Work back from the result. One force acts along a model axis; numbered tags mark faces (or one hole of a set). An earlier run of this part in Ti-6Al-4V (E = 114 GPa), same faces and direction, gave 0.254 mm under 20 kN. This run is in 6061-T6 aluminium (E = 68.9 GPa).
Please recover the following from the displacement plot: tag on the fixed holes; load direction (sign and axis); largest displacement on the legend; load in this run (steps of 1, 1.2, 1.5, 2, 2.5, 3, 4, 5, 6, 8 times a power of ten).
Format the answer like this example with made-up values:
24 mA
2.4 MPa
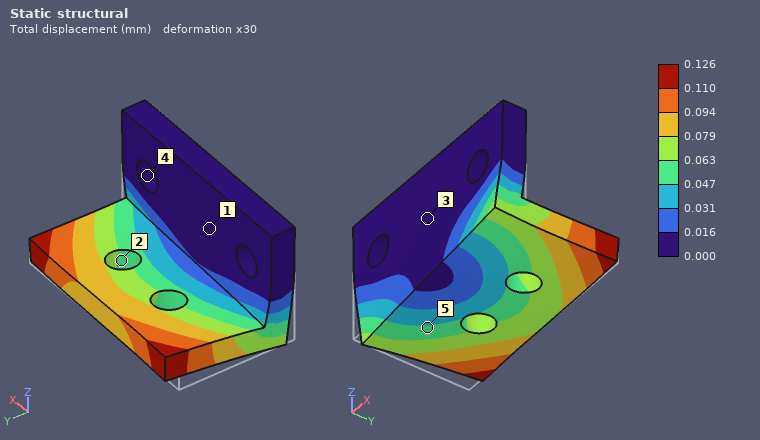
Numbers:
4
+X
0.126 mm
6 kN
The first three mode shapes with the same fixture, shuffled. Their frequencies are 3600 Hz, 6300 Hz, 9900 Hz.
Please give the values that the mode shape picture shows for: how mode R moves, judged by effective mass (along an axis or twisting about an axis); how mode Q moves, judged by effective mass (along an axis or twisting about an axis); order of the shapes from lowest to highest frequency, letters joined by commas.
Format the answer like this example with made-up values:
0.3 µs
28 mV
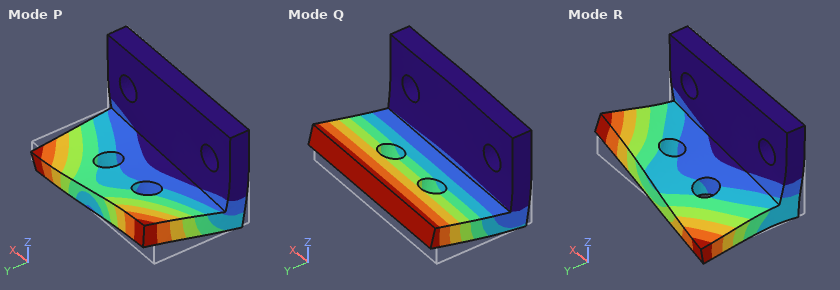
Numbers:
along X
along Z
Q, P, R
